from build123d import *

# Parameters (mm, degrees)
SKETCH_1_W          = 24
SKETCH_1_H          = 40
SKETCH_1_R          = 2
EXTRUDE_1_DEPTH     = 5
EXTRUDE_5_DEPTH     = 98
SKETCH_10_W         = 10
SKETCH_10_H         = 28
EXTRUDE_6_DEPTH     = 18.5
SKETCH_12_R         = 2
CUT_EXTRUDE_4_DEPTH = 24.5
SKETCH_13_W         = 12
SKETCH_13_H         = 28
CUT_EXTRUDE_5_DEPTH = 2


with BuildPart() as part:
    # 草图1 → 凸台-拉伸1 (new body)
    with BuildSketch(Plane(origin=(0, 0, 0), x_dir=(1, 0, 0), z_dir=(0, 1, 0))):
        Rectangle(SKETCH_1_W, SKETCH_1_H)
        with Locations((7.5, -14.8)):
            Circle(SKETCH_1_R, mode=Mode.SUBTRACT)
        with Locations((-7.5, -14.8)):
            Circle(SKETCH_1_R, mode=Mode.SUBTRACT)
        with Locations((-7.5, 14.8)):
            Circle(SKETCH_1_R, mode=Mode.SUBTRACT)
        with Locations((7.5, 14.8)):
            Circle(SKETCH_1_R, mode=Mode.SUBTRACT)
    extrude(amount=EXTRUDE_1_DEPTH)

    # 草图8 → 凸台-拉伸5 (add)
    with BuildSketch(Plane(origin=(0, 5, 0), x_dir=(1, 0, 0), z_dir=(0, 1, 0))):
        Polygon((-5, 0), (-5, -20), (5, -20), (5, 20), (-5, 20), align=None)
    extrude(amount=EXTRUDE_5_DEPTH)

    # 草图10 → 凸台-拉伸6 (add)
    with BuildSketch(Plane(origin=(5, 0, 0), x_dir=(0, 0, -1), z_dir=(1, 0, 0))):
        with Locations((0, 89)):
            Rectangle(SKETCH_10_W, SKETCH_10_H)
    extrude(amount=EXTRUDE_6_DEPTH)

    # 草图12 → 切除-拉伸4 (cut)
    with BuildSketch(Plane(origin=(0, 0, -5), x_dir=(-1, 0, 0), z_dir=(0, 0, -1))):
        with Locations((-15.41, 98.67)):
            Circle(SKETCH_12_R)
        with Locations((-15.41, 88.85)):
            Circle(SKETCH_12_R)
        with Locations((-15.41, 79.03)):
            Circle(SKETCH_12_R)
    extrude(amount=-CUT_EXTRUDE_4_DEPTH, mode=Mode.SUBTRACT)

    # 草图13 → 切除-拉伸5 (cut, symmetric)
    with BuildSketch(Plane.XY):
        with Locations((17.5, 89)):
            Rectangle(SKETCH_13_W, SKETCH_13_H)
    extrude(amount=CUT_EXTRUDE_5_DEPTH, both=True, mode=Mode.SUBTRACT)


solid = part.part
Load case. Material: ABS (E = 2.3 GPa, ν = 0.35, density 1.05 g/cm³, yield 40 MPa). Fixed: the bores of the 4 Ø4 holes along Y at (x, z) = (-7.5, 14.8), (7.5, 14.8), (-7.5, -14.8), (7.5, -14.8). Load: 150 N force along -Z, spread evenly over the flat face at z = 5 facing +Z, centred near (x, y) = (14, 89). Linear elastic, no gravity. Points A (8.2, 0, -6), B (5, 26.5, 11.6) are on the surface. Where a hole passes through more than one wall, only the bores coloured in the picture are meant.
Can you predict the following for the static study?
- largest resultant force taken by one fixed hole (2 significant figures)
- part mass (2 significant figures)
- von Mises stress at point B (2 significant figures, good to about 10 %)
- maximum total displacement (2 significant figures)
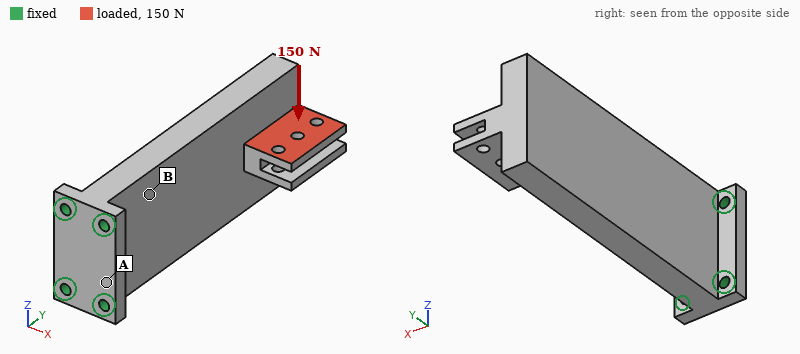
280 N
50 g
3.9 MPa
1.2 mm
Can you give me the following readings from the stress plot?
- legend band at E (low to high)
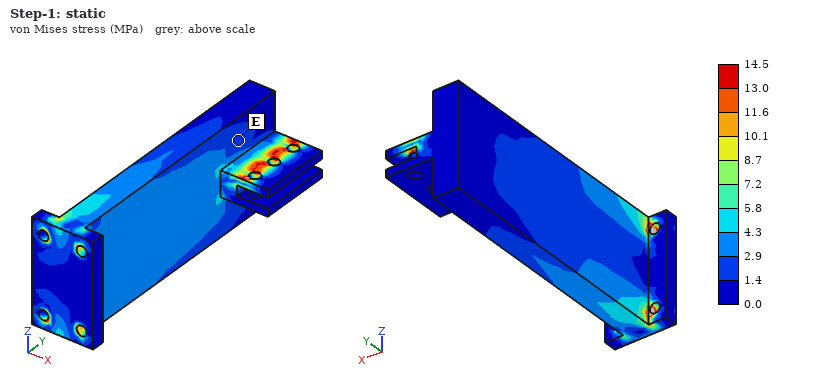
1.4 to 2.9 MPa
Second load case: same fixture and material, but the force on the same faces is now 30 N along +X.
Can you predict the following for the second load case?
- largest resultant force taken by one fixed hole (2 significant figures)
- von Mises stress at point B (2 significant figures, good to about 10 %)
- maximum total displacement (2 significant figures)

100 N
2.8 MPa
1.2 mm
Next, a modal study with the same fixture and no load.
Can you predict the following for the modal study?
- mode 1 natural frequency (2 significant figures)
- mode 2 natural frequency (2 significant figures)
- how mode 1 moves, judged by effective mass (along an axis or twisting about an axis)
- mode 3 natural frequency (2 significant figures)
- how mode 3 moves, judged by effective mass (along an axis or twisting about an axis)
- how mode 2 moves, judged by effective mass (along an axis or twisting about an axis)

200 Hz
660 Hz
along X
1000 Hz
twisting about Y
along Z
